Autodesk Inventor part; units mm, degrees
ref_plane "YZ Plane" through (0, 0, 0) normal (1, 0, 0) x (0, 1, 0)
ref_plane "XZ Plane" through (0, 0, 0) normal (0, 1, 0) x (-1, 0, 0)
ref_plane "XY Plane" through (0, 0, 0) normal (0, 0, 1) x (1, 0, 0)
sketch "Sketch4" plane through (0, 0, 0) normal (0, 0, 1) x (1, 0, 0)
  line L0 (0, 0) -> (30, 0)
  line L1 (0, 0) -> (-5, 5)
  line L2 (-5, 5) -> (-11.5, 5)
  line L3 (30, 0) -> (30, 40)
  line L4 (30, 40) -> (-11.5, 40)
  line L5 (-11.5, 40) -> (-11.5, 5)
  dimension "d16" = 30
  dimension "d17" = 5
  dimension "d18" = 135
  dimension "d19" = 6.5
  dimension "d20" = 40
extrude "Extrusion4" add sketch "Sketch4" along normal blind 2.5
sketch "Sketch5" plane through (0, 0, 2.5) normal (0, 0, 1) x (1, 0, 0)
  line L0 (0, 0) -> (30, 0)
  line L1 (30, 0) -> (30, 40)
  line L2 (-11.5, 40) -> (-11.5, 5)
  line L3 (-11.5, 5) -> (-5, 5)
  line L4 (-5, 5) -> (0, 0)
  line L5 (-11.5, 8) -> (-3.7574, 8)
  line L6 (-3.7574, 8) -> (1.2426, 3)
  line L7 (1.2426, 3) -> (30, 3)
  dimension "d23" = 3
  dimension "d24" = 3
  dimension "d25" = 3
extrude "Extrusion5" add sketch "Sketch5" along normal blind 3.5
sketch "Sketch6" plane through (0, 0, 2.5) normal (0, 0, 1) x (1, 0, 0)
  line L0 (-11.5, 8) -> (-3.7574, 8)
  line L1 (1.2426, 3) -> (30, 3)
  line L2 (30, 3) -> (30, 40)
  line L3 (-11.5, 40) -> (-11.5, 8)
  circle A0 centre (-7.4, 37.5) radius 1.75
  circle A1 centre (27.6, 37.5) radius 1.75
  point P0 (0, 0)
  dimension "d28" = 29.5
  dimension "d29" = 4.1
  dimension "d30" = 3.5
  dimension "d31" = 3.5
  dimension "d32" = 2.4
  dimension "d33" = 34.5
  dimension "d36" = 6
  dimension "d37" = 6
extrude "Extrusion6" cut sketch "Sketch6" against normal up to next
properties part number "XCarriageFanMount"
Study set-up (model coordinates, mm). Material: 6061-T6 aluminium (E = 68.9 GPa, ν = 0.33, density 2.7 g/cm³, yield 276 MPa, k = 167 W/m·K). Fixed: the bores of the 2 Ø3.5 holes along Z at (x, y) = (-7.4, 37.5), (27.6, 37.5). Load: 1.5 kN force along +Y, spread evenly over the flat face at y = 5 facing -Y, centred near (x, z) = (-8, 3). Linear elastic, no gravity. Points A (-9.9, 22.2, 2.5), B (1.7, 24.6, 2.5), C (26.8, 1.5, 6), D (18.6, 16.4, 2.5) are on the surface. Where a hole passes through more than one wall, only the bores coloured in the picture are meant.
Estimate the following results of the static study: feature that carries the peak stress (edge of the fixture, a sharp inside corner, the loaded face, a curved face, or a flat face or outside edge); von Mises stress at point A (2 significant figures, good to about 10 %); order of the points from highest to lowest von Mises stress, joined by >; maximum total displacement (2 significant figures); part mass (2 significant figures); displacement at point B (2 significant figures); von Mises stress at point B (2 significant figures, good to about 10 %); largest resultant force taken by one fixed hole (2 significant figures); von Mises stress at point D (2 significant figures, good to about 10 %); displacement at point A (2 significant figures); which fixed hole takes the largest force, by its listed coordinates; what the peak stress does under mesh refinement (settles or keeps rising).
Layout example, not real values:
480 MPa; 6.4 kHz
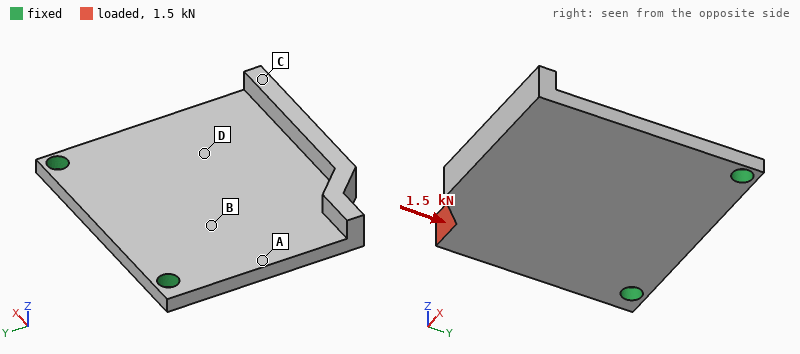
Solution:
edge of the fixture; 140 MPa; A > B > D > C; 0.61 mm; 12 g; 0.097 mm; 75 MPa; 1.5 kN; 41 MPa; 0.11 mm; (-7.4, 37.5); keeps rising
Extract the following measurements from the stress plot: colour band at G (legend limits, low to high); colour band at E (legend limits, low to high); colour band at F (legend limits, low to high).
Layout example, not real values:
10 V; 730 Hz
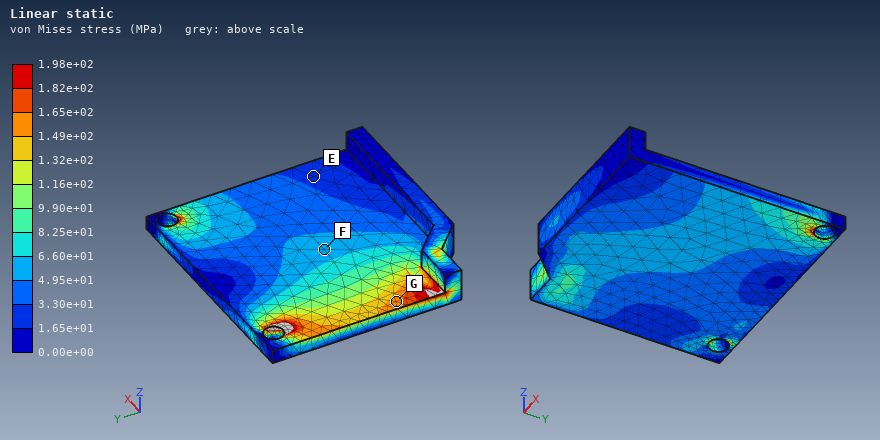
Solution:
1.49e+02 to 1.65e+02 MPa; 1.65e+01 to 3.30e+01 MPa; 4.95e+01 to 6.60e+01 MPa
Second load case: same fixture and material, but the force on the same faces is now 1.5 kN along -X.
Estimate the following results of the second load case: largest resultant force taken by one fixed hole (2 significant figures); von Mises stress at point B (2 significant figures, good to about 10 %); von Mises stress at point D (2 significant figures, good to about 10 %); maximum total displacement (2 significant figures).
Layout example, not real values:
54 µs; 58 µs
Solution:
1.6 kN; 69 MPa; 64 MPa; 0.23 mm
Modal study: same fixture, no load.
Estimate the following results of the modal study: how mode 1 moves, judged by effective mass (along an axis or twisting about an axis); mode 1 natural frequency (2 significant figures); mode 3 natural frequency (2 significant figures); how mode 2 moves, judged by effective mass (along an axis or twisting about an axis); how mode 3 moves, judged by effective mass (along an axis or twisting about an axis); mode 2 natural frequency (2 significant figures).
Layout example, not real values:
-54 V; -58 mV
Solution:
along Z; 1100 Hz; 7300 Hz; twisting about Y; along Z; 3300 Hz
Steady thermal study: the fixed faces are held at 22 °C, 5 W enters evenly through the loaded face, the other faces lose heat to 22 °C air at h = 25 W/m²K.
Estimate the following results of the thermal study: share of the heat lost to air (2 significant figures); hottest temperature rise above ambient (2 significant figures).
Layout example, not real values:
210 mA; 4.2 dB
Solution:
12 %; 18 K
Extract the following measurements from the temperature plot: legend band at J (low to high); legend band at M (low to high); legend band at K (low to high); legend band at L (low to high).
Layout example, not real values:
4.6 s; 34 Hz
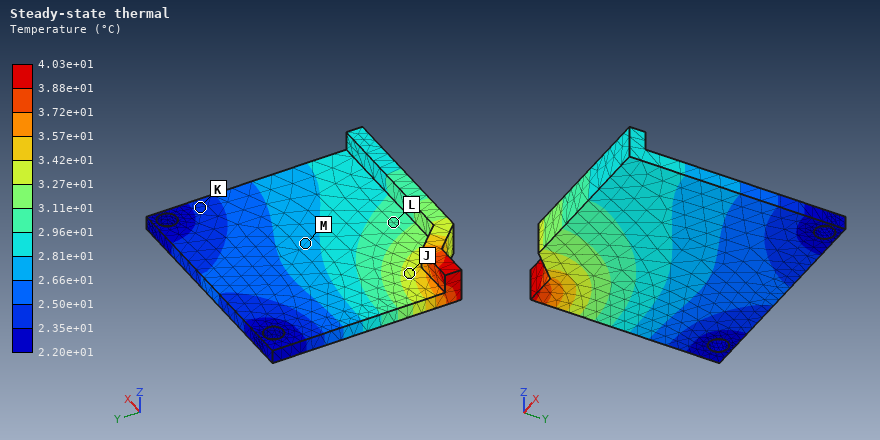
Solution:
3.27e+01 to 3.42e+01 °C; 2.66e+01 to 2.81e+01 °C; 2.35e+01 to 2.50e+01 °C; 2.96e+01 to 3.11e+01 °C
